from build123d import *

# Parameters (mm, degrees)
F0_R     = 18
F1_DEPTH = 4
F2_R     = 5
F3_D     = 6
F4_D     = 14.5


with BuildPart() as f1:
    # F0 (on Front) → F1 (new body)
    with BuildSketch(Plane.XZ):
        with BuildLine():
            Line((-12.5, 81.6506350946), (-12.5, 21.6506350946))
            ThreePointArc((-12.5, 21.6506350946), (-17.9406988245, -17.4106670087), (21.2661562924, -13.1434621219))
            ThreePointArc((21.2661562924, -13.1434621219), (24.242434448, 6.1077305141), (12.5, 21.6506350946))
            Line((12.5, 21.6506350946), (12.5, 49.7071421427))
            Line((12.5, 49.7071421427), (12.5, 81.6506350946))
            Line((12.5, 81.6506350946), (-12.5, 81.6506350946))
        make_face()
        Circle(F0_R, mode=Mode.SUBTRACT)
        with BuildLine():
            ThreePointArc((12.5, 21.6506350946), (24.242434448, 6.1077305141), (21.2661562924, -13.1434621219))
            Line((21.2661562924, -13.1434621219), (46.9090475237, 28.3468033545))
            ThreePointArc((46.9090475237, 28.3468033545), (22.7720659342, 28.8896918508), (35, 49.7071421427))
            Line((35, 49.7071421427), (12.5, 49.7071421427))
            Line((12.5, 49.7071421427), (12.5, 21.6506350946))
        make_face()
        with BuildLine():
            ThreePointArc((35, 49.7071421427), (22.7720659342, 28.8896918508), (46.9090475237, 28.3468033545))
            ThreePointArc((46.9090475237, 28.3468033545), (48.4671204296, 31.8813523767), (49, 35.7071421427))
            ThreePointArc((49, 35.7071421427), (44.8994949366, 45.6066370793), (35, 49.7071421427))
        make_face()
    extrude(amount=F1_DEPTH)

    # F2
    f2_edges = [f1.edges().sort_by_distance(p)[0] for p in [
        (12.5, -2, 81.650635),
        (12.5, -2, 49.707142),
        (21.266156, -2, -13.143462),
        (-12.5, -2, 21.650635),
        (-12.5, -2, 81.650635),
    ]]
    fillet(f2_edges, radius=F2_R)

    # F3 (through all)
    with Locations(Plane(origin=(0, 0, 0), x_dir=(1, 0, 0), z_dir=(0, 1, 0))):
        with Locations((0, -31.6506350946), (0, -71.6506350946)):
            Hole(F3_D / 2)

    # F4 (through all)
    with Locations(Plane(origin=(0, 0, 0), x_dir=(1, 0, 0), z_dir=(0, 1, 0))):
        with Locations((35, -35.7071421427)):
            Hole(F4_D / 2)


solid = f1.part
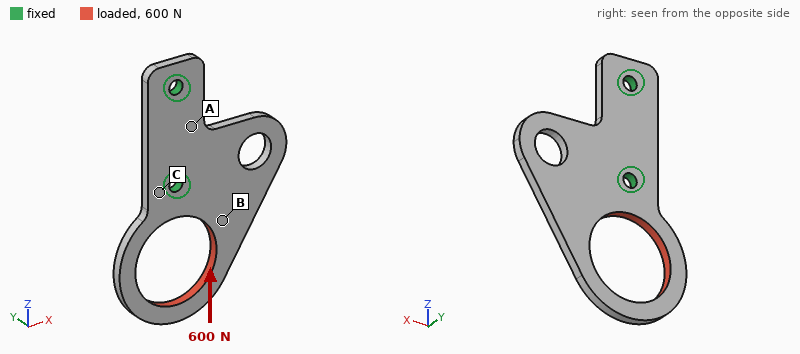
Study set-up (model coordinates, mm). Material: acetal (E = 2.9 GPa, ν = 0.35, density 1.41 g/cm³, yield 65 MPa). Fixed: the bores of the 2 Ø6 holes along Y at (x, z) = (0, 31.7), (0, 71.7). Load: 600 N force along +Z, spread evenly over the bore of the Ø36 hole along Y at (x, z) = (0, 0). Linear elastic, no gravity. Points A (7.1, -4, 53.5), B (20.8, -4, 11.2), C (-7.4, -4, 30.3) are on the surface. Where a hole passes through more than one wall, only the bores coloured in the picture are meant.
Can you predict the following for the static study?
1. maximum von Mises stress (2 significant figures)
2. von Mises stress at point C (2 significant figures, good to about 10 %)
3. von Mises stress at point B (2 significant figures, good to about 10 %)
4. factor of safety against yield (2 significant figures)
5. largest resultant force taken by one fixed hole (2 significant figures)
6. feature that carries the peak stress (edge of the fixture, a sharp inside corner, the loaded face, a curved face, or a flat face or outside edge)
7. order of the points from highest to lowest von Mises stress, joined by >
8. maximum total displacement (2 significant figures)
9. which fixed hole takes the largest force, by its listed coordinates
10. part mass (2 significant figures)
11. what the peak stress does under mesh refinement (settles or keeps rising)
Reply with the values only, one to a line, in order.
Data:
55 MPa
9.1 MPa
5.5 MPa
1.2
480 N
a curved face
C > B > A
0.78 mm
(0, 31.7)
19 g
settles
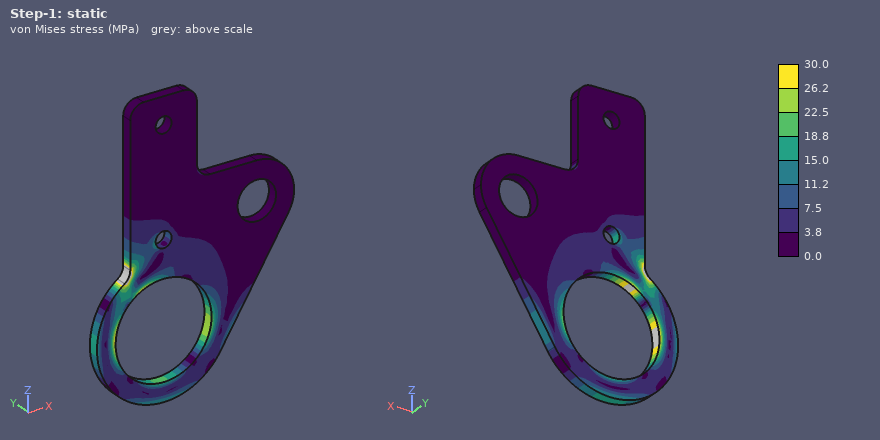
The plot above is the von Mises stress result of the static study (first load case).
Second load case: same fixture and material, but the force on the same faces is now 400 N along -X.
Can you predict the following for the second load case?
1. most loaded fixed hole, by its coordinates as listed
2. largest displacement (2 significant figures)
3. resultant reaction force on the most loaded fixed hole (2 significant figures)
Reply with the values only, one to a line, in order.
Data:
(0, 31.7)
1.3 mm
660 N
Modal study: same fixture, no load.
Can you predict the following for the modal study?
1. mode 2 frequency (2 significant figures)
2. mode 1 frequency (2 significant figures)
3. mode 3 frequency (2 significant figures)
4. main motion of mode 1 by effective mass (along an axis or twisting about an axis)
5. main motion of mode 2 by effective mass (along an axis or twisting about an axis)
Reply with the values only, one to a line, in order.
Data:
450 Hz
310 Hz
720 Hz
along Y
along Y
